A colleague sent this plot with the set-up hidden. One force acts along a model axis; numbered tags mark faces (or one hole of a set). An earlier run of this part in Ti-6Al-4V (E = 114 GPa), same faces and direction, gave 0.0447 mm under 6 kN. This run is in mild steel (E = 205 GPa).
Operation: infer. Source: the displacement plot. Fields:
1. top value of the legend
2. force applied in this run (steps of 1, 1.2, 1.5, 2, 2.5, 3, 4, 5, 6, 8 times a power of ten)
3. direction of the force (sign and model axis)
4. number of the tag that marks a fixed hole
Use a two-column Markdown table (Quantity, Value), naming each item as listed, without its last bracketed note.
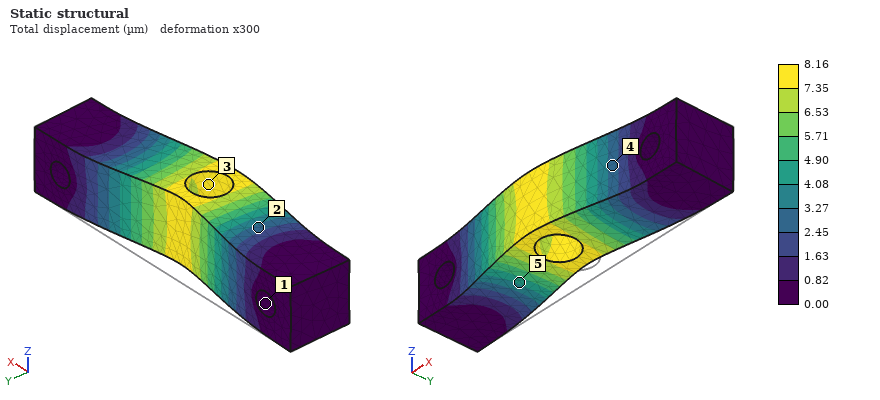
| Quantity | Value |
|---|---|
| top value of the legend | 8.16 µm |
| force applied in this run | 2 kN |
| direction of the force | -Y |
| number of the tag that marks a fixed hole | 1 |
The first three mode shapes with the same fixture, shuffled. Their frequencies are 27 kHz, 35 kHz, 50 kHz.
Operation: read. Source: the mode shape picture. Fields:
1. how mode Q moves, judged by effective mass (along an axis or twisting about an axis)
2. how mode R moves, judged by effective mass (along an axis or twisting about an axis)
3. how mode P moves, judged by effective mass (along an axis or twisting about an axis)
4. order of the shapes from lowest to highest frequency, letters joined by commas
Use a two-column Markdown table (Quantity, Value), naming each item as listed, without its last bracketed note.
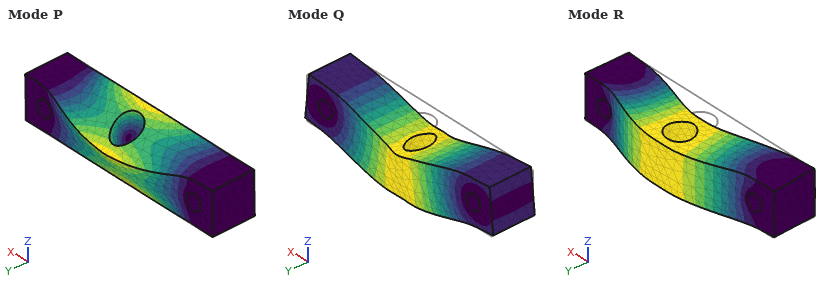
| Quantity | Value |
|---|---|
| how mode Q moves, judged by effective mass | along Z |
| how mode R moves, judged by effective mass | along Y |
| how mode P moves, judged by effective mass | twisting about X |
| order of the shapes from lowest to highest frequency, letters joined by commas | Q, R, P |
